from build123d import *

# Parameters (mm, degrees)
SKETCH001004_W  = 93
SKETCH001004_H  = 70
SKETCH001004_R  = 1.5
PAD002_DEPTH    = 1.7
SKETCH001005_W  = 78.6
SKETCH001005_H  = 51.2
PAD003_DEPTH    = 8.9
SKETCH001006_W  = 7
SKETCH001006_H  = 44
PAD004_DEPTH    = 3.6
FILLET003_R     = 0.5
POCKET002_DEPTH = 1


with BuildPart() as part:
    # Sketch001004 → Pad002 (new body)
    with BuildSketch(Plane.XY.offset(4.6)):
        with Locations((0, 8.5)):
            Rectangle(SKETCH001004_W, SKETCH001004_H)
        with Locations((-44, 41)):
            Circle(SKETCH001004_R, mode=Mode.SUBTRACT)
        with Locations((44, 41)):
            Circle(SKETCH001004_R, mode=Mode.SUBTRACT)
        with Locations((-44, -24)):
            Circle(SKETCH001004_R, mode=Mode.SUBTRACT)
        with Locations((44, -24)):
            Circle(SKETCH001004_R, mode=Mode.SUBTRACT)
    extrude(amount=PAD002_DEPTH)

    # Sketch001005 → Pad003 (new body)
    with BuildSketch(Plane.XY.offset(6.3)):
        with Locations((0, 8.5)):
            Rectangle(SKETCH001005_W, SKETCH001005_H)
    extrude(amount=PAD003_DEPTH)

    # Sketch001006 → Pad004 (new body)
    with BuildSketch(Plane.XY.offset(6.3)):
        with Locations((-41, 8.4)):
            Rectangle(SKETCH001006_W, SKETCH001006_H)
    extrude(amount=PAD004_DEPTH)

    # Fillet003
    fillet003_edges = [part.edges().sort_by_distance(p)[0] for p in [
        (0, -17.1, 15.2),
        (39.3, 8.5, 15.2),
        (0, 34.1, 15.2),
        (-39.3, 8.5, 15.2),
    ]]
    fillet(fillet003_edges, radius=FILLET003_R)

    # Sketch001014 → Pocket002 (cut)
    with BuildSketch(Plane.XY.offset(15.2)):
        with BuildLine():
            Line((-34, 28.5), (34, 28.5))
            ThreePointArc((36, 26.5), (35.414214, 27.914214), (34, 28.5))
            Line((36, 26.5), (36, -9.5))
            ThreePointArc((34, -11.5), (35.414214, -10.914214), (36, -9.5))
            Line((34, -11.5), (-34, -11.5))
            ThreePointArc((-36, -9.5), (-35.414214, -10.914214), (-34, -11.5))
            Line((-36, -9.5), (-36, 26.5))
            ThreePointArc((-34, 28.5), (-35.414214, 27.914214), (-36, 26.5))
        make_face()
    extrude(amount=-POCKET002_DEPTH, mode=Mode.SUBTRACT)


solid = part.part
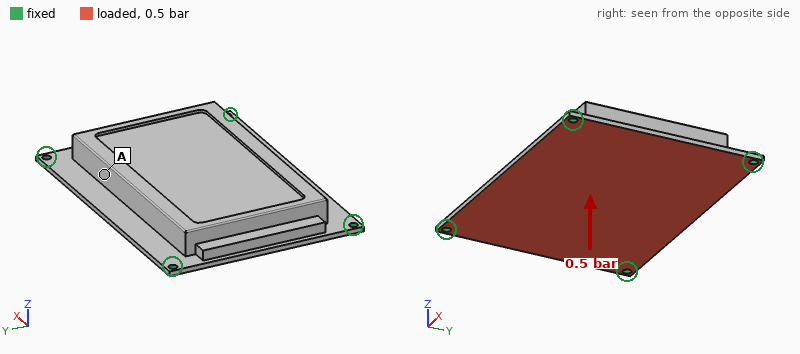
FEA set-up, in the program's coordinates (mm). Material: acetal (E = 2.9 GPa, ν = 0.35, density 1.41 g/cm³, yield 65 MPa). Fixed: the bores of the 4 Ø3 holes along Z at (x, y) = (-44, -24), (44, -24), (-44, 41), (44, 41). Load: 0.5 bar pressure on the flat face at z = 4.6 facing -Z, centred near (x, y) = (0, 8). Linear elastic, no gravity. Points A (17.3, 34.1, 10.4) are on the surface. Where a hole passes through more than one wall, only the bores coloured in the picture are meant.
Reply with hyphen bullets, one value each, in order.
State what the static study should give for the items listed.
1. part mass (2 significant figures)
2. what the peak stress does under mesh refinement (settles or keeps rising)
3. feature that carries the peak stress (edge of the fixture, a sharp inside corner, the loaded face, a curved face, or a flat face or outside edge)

- 63 g
- keeps rising
- edge of the fixture
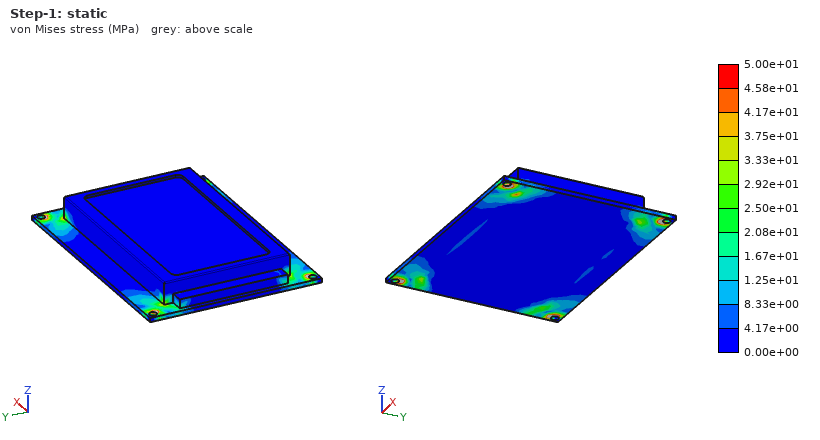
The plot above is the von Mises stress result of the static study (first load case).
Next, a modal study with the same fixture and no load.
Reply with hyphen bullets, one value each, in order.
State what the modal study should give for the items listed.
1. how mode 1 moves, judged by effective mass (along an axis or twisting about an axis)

- along Z
